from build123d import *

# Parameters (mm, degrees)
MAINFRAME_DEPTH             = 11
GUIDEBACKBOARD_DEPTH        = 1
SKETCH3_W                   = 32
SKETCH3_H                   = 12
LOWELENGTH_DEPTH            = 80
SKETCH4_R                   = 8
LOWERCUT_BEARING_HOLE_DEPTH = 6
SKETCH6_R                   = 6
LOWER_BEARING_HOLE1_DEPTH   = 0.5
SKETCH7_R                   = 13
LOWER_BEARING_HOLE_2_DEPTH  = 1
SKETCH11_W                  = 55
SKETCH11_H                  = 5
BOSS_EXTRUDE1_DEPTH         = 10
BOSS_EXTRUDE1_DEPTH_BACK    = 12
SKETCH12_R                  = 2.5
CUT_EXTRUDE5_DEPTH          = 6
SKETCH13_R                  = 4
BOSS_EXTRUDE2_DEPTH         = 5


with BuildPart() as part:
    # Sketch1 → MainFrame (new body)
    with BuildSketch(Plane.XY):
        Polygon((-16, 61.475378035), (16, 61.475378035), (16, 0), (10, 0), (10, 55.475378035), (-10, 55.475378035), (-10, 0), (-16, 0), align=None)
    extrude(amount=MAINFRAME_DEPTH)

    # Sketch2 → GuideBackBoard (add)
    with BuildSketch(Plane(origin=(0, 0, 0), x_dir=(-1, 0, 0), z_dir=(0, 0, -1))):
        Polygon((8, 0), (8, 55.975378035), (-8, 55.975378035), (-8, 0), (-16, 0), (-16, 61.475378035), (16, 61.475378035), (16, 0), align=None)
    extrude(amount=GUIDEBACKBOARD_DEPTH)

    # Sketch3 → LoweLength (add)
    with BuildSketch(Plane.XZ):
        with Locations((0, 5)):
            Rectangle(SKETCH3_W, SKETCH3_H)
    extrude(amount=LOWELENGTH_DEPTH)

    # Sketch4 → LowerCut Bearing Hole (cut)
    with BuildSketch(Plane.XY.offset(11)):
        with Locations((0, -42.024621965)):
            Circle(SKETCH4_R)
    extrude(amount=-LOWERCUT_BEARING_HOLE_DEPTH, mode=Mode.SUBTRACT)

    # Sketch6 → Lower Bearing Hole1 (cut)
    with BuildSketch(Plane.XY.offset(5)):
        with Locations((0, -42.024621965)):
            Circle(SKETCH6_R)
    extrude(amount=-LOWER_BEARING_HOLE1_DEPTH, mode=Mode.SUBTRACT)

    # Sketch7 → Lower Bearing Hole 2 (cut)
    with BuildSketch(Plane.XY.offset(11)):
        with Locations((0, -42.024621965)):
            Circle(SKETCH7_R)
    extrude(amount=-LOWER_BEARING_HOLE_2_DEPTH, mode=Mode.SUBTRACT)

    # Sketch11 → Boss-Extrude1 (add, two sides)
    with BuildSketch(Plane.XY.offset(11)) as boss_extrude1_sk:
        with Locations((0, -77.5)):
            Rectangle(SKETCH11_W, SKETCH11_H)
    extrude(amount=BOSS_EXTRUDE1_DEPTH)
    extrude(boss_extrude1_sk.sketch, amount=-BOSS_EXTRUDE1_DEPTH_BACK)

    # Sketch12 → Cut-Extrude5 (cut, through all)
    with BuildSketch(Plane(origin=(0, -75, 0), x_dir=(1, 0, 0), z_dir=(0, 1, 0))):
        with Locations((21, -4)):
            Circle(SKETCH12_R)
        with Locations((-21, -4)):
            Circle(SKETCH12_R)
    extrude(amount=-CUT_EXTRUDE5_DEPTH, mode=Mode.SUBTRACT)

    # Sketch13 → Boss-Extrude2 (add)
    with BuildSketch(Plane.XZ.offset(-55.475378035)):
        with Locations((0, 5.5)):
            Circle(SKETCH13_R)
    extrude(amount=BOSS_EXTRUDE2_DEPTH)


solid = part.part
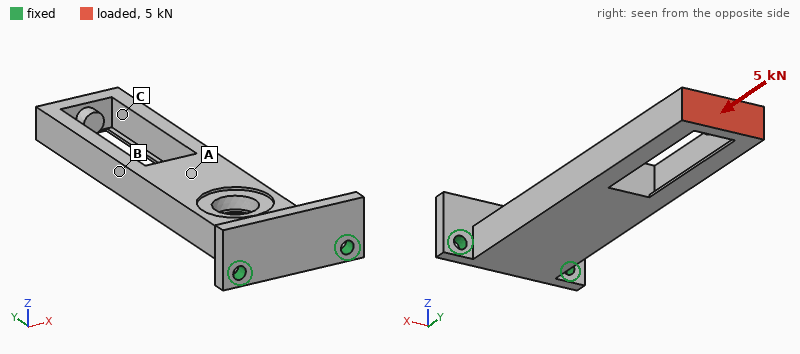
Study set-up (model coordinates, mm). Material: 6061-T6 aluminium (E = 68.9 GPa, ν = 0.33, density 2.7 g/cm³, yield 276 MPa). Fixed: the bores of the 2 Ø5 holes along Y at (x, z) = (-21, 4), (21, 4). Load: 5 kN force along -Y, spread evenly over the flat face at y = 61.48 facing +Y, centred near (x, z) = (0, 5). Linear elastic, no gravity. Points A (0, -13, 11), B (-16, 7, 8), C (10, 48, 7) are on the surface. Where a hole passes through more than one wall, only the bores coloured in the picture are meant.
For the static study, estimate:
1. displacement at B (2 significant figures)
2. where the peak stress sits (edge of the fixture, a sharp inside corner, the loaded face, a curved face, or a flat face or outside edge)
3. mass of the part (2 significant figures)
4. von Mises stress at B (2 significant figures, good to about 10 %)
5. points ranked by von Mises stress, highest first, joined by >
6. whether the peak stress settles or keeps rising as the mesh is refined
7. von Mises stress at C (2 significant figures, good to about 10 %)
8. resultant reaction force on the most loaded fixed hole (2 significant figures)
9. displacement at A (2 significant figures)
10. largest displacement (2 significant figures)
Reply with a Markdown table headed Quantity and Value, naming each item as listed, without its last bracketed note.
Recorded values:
| Quantity | Value |
|---|---|
| displacement at B | 0.072 mm |
| where the peak stress sits | edge of the fixture |
| mass of the part | 120 g |
| von Mises stress at B | 42 MPa |
| points ranked by von Mises stress, highest first, joined by > | C > B > A |
| whether the peak stress settles or keeps rising as the mesh is refined | keeps rising |
| von Mises stress at C | 72 MPa |
| resultant reaction force on the most loaded fixed hole | 2.7 kN |
| displacement at A | 0.050 mm |
| largest displacement | 0.16 mm |
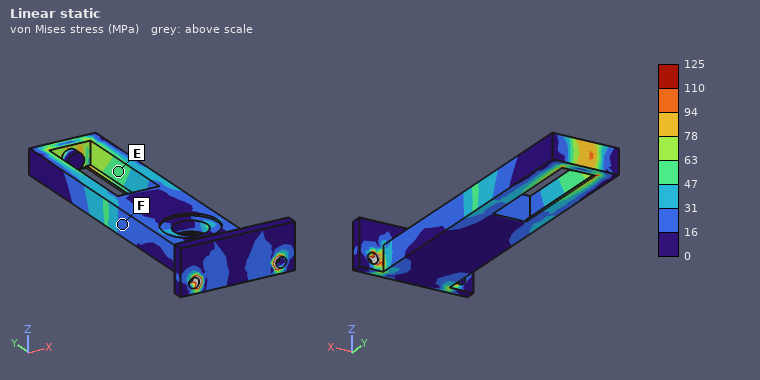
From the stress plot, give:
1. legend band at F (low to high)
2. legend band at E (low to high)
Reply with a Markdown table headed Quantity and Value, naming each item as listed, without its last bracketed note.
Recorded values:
| Quantity | Value |
|---|---|
| legend band at F | 16 to 31 MPa |
| legend band at E | 47 to 63 MPa |
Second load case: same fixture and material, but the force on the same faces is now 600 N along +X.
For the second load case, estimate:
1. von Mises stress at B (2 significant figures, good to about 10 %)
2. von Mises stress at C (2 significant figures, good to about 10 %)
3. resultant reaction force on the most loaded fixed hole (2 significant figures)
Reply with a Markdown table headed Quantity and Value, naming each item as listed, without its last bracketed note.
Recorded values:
| Quantity | Value |
|---|---|
| von Mises stress at B | 93 MPa |
| von Mises stress at C | 79 MPa |
| resultant reaction force on the most loaded fixed hole | 2.4 kN |
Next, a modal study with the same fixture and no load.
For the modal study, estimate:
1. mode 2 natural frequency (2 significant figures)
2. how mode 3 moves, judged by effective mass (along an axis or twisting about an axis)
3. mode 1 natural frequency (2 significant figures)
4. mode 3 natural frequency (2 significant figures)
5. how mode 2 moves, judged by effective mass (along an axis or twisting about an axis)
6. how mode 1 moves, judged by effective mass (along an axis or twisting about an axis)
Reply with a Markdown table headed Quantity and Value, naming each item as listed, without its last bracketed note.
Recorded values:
| Quantity | Value |
|---|---|
| mode 2 natural frequency | 1100 Hz |
| how mode 3 moves, judged by effective mass | along Z |
| mode 1 natural frequency | 400 Hz |
| mode 3 natural frequency | 2200 Hz |
| how mode 2 moves, judged by effective mass | along X |
| how mode 1 moves, judged by effective mass | along Z |
